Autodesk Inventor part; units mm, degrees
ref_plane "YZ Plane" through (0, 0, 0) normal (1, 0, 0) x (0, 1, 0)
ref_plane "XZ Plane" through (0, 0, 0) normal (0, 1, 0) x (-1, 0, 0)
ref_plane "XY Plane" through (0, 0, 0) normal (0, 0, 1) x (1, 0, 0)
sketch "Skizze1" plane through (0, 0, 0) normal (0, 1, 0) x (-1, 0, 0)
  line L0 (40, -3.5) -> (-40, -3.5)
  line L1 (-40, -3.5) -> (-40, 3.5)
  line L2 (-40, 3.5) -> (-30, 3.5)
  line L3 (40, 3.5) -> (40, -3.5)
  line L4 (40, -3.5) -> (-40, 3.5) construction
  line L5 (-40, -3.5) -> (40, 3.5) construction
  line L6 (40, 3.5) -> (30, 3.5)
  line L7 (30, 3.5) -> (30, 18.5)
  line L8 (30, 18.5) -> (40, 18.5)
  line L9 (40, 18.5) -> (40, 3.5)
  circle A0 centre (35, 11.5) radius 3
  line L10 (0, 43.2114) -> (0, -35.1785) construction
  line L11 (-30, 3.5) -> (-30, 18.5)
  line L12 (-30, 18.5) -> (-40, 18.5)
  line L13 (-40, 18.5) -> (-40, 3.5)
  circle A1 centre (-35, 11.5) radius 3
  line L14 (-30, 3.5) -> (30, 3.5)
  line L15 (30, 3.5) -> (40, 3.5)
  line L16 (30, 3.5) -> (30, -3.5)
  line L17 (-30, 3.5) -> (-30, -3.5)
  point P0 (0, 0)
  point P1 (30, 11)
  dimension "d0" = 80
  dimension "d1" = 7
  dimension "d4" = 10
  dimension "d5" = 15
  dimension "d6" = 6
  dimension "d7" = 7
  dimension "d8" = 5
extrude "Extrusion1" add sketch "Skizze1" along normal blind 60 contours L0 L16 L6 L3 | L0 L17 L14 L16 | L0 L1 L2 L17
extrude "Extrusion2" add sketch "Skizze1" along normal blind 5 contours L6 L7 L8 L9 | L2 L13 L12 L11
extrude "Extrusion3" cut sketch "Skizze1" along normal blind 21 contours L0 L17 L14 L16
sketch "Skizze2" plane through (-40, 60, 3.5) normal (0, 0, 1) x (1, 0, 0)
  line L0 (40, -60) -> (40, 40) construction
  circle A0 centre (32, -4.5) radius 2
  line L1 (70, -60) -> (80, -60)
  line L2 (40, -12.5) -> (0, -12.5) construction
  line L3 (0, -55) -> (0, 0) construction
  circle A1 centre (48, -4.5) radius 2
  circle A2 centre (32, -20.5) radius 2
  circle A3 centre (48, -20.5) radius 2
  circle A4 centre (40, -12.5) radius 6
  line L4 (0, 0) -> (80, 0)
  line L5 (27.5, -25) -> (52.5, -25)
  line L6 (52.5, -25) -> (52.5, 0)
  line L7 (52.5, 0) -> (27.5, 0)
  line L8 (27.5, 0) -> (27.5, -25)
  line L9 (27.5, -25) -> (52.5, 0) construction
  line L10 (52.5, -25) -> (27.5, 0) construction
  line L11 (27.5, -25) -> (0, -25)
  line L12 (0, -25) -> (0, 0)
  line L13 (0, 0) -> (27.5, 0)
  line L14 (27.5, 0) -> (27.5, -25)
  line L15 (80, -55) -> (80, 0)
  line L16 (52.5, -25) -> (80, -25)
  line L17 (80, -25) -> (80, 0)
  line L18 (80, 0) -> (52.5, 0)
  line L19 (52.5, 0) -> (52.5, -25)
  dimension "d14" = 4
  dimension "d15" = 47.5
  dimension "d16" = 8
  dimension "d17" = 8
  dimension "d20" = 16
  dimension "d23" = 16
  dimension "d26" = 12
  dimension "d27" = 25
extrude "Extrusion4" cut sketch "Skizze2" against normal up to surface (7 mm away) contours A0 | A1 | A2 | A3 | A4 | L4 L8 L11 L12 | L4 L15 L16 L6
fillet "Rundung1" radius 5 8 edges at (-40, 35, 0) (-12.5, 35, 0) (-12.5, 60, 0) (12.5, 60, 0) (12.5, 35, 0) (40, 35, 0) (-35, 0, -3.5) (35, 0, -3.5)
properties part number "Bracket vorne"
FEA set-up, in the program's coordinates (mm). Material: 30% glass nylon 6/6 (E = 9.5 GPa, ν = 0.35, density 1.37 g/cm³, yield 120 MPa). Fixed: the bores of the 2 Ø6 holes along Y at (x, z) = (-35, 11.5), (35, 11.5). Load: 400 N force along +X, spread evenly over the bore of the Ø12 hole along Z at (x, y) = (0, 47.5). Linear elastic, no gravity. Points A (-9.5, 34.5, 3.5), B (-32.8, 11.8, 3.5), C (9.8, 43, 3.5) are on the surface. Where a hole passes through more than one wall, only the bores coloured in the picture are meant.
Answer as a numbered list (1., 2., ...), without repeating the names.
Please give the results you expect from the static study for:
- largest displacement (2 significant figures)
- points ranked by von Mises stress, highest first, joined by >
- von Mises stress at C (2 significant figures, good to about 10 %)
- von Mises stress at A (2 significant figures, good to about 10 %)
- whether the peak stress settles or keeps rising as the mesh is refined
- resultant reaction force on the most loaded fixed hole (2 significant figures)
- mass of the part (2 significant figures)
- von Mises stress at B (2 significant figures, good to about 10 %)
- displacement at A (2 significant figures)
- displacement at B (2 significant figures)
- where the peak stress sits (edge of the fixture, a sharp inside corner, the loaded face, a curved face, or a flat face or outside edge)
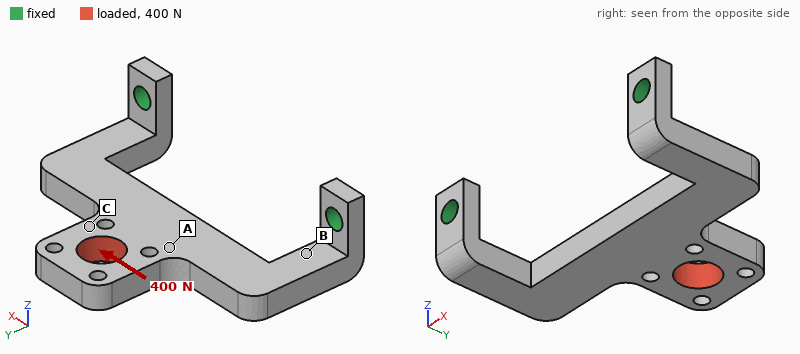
1. 0.29 mm
2. B > C > A
3. 7.5 MPa
4. 4.3 MPa
5. keeps rising
6. 300 N
7. 21 g
8. 16 MPa
9. 0.22 mm
10. 0.11 mm
11. edge of the fixture
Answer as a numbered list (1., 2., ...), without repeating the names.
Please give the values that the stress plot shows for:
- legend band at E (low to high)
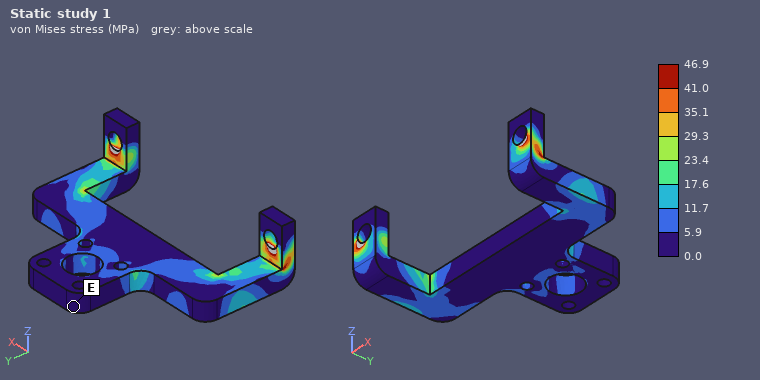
1. 0.0 to 5.9 MPa
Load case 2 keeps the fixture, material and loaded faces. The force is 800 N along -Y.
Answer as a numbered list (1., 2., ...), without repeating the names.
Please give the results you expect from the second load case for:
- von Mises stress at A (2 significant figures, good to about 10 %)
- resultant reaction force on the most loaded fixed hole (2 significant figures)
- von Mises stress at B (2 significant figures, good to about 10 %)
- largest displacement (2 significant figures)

1. 13 MPa
2. 430 N
3. 12 MPa
4. 1.1 mm
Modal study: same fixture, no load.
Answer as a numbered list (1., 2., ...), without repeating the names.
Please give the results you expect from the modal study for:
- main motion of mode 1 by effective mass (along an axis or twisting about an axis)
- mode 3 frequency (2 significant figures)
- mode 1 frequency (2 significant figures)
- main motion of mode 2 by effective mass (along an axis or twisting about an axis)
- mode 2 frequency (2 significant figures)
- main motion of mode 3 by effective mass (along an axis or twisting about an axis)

1. along Z
2. 2000 Hz
3. 480 Hz
4. along X
5. 1600 Hz
6. along X
